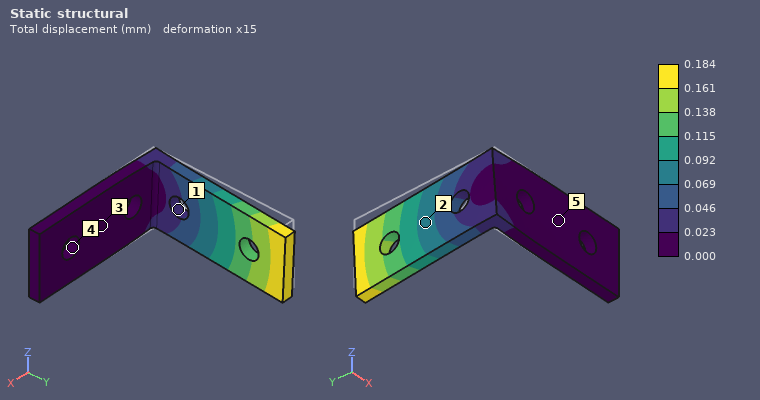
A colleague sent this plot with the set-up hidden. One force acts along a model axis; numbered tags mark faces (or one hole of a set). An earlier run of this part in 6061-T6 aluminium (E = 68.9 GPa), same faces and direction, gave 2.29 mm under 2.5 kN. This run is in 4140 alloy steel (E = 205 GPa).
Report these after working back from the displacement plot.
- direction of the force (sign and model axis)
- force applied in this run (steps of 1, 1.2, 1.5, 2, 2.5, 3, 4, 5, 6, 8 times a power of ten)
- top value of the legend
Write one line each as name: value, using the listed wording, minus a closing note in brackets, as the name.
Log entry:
direction of the force: -Z
force applied in this run: 600 N
top value of the legend: 0.184 mm
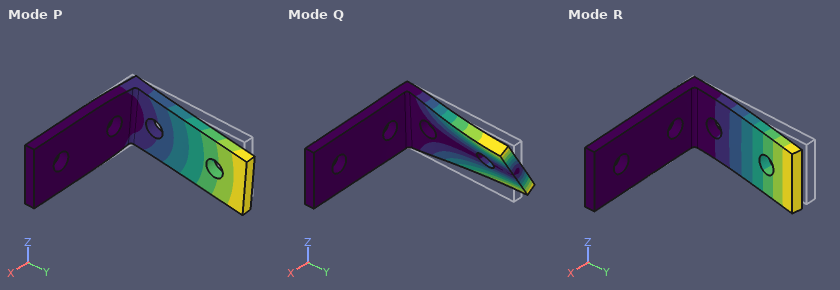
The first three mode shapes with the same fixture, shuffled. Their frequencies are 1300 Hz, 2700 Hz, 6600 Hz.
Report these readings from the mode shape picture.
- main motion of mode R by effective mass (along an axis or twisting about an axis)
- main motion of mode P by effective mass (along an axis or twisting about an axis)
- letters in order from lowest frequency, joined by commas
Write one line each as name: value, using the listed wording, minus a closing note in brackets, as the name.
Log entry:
main motion of mode R by effective mass: along X
main motion of mode P by effective mass: along Z
letters in order from lowest frequency, joined by commas: R, P, Q
